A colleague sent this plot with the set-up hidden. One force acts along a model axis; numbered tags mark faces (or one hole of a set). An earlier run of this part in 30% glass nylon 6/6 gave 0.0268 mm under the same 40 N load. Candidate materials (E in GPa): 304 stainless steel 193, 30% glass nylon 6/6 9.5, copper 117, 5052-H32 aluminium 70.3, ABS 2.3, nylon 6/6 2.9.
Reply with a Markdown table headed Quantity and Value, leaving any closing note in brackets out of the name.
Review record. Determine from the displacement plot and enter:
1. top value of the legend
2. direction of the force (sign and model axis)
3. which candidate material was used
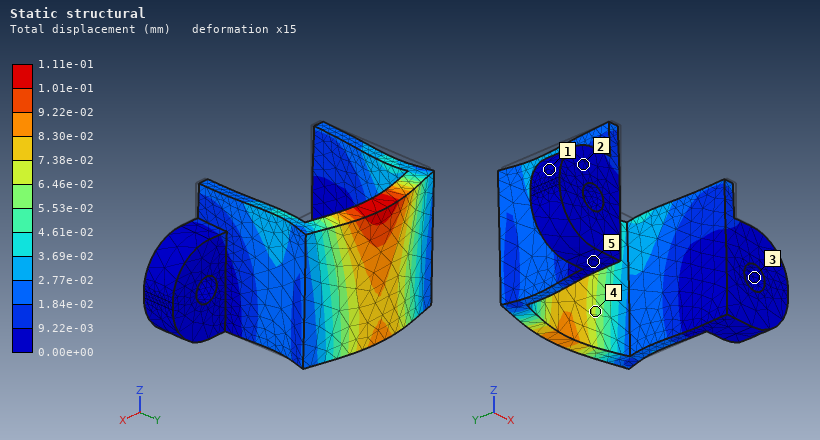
| Quantity | Value |
|---|---|
| top value of the legend | 1.11e-01 mm |
| direction of the force | +Y |
| which candidate material was used | ABS |
